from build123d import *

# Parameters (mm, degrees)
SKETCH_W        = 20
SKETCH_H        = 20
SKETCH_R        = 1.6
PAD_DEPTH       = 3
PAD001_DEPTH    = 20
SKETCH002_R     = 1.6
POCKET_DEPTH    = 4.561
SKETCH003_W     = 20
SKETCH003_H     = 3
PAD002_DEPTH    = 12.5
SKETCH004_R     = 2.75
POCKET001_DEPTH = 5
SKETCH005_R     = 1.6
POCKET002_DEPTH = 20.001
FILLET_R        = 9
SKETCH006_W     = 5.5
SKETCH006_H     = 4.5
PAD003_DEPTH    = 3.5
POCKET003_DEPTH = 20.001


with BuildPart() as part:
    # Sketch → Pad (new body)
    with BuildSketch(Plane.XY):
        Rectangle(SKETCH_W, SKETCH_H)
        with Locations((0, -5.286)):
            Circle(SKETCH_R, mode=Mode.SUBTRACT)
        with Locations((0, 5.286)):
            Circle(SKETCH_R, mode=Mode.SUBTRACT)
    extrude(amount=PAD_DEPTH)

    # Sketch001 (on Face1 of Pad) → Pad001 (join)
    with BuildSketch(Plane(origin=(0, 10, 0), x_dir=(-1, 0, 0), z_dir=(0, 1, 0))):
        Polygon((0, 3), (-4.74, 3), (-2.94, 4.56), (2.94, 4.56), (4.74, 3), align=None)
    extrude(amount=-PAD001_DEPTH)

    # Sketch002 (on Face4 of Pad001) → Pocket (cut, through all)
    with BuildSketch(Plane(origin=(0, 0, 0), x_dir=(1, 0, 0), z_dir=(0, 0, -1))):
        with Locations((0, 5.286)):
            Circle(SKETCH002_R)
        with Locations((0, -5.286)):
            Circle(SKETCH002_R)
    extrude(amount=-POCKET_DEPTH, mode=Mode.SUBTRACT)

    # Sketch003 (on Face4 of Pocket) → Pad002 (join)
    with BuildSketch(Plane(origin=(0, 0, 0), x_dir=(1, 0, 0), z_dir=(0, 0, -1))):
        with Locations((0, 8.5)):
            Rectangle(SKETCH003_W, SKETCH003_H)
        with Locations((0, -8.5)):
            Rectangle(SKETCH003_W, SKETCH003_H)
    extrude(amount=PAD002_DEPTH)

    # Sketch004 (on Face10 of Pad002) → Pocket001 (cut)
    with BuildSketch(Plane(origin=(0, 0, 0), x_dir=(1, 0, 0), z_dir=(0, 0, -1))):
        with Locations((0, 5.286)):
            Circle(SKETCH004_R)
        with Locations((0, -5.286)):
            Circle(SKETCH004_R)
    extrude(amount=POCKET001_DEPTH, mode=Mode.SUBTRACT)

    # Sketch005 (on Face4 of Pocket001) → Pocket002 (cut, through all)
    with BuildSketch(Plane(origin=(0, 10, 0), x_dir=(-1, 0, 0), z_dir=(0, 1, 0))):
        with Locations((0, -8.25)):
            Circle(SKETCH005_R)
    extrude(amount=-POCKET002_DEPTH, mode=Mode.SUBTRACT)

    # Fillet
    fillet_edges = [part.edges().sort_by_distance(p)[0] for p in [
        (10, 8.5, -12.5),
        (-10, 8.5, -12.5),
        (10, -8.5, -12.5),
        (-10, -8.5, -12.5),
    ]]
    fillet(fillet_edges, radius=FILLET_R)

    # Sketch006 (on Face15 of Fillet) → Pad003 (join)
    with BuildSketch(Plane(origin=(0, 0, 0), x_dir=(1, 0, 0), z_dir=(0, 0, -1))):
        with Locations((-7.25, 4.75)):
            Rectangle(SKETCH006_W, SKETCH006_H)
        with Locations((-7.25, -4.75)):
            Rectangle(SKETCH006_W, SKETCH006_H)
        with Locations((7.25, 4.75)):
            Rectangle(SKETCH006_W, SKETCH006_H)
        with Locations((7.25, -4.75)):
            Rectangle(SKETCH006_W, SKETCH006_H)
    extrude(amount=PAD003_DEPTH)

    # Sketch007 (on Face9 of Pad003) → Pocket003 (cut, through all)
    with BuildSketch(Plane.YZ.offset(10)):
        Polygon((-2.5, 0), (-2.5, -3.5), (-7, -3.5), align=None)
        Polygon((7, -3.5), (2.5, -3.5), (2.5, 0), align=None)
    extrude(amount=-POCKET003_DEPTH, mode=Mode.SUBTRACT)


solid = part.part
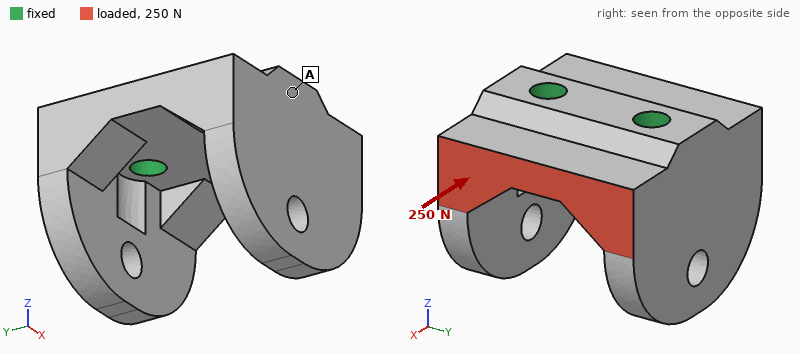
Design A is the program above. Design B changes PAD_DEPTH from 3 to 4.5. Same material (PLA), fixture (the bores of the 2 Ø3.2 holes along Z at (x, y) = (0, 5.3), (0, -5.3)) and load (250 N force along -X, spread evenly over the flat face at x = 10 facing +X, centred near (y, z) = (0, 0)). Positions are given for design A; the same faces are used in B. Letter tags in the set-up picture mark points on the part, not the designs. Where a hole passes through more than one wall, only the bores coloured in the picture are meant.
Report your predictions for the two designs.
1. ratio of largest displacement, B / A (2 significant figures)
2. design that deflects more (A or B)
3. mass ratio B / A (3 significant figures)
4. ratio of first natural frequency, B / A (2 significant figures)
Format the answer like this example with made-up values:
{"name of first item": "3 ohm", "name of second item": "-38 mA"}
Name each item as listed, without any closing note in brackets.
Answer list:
{"ratio of largest displacement, B / A": "0.60", "design that deflects more": "A", "mass ratio B / A": "1.13", "ratio of first natural frequency, B / A": "1.1"}
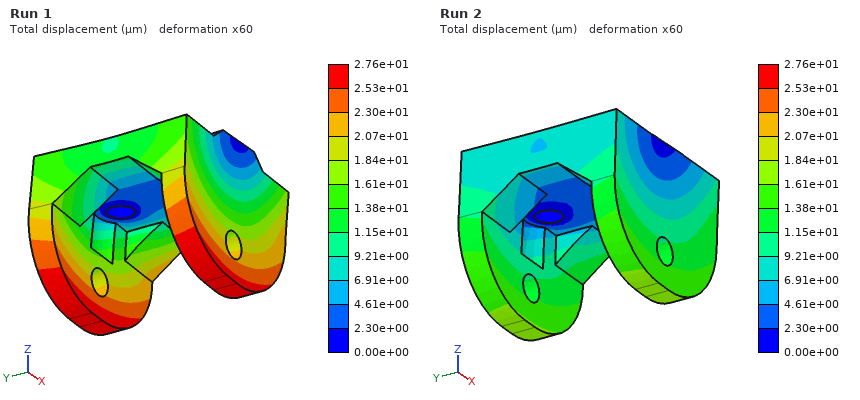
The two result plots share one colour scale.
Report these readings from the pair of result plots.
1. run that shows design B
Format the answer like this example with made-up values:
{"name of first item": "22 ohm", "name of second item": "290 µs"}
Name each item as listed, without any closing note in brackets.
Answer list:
{"run that shows design B": "Run 2"}
